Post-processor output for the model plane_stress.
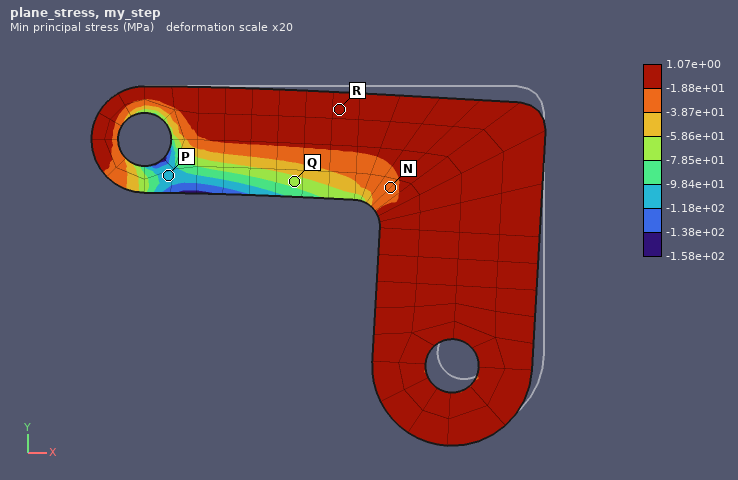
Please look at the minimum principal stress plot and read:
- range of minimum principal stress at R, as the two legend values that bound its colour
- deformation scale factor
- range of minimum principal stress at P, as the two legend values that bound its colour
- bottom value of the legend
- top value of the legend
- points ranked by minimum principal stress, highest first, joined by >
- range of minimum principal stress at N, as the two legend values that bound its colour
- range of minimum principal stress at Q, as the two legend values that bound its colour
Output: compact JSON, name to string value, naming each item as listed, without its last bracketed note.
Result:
{"range of minimum principal stress at R, as the two legend values that bound its colour": "-1.88e+01 to 1.07e+00 MPa", "deformation scale factor": "20", "range of minimum principal stress at P, as the two legend values that bound its colour": "-1.18e+02 to -9.84e+01 MPa", "bottom value of the legend": "-1.58e+02 MPa", "top value of the legend": "1.07e+00 MPa", "points ranked by minimum principal stress, highest first, joined by >": "R > N > Q > P", "range of minimum principal stress at N, as the two legend values that bound its colour": "-3.87e+01 to -1.88e+01 MPa", "range of minimum principal stress at Q, as the two legend values that bound its colour": "-7.85e+01 to -5.86e+01 MPa"}
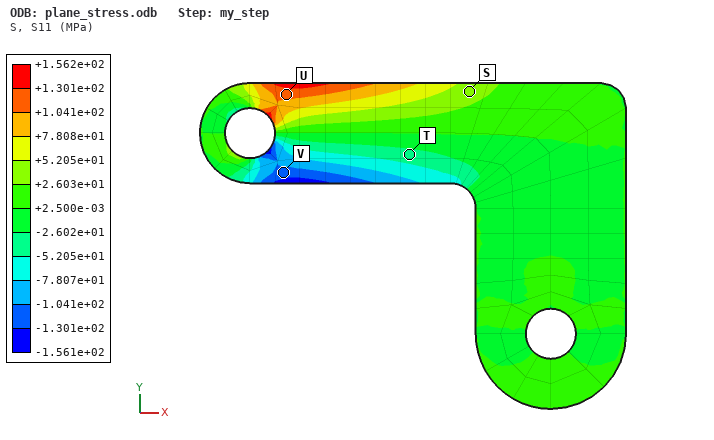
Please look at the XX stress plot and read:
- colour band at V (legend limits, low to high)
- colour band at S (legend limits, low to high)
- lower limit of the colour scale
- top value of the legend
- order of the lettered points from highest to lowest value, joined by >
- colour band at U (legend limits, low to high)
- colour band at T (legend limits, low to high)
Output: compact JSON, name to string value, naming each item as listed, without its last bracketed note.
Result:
{"colour band at V": "-1.301e+02 to -1.041e+02 MPa", "colour band at S": "+2.603e+01 to +5.205e+01 MPa", "lower limit of the colour scale": "-1.561e+02 MPa", "top value of the legend": "+1.562e+02 MPa", "order of the lettered points from highest to lowest value, joined by >": "U > S > T > V", "colour band at U": "+1.041e+02 to +1.301e+02 MPa", "colour band at T": "-5.205e+01 to -2.602e+01 MPa"}
